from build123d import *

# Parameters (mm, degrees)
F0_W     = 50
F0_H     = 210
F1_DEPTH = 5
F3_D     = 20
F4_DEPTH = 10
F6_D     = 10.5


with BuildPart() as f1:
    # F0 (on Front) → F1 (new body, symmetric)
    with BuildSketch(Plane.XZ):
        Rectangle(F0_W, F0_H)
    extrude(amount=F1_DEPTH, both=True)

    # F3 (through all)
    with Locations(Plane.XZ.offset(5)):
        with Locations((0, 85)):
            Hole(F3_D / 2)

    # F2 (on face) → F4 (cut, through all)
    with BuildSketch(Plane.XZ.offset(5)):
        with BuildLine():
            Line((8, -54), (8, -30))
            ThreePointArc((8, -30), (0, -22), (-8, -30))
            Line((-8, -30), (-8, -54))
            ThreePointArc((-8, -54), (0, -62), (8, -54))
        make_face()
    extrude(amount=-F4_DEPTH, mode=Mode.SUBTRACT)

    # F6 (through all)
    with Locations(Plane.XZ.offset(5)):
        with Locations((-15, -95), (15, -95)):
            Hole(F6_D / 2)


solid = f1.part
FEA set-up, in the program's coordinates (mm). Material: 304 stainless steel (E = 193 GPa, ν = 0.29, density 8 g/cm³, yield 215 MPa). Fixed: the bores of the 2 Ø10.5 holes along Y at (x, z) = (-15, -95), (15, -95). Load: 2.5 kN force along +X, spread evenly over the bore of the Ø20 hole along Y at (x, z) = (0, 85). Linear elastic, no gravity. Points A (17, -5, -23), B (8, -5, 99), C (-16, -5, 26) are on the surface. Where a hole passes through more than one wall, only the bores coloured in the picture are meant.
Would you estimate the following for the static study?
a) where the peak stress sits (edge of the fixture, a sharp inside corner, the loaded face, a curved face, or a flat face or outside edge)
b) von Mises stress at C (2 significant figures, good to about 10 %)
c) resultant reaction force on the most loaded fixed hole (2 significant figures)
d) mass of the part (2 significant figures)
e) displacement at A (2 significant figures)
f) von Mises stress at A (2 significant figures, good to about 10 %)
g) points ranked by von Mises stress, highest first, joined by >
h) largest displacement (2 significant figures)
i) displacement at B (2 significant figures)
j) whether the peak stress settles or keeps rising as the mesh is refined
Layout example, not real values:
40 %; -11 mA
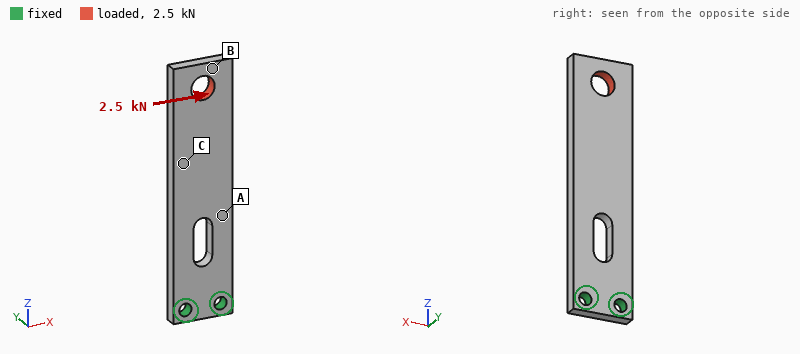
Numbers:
edge of the fixture; 24 MPa; 13 kN; 750 g; 0.071 mm; 44 MPa; A > C > B; 0.31 mm; 0.30 mm; keeps rising
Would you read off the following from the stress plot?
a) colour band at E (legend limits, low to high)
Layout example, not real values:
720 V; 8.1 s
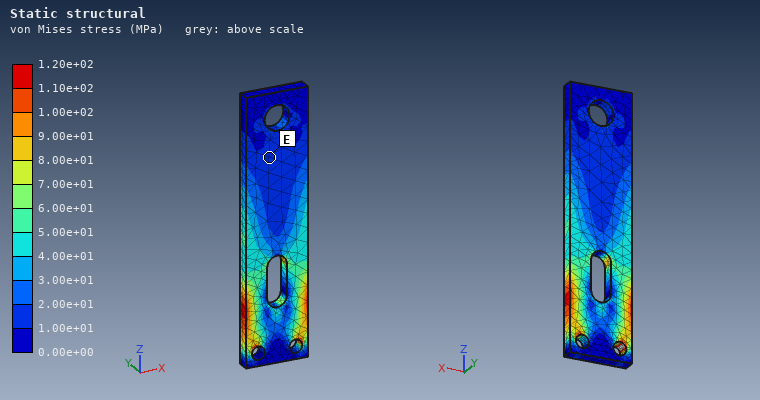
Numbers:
1.00e+01 to 2.00e+01 MPa
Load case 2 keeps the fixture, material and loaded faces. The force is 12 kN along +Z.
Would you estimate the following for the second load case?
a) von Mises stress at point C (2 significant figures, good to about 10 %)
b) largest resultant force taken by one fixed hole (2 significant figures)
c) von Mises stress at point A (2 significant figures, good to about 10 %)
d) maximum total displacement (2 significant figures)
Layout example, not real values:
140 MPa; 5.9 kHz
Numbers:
24 MPa; 6.0 kN; 33 MPa; 32 µm
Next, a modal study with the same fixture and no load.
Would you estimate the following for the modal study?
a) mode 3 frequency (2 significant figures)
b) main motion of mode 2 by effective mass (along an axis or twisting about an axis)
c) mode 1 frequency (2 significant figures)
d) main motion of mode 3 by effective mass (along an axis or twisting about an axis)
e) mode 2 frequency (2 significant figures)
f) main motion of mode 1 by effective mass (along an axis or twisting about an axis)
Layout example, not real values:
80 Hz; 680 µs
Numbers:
1300 Hz; along X; 200 Hz; along Y; 960 Hz; along Y
